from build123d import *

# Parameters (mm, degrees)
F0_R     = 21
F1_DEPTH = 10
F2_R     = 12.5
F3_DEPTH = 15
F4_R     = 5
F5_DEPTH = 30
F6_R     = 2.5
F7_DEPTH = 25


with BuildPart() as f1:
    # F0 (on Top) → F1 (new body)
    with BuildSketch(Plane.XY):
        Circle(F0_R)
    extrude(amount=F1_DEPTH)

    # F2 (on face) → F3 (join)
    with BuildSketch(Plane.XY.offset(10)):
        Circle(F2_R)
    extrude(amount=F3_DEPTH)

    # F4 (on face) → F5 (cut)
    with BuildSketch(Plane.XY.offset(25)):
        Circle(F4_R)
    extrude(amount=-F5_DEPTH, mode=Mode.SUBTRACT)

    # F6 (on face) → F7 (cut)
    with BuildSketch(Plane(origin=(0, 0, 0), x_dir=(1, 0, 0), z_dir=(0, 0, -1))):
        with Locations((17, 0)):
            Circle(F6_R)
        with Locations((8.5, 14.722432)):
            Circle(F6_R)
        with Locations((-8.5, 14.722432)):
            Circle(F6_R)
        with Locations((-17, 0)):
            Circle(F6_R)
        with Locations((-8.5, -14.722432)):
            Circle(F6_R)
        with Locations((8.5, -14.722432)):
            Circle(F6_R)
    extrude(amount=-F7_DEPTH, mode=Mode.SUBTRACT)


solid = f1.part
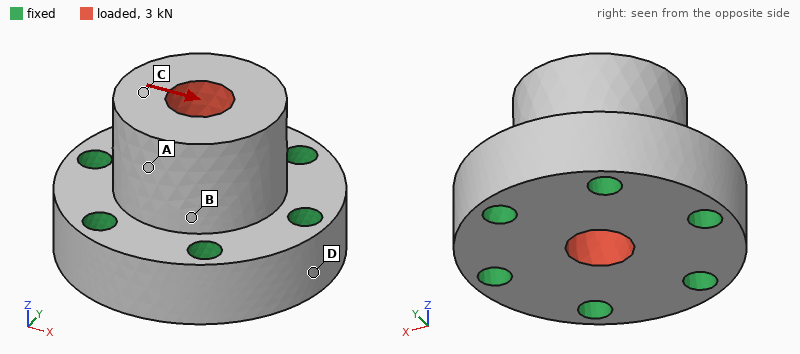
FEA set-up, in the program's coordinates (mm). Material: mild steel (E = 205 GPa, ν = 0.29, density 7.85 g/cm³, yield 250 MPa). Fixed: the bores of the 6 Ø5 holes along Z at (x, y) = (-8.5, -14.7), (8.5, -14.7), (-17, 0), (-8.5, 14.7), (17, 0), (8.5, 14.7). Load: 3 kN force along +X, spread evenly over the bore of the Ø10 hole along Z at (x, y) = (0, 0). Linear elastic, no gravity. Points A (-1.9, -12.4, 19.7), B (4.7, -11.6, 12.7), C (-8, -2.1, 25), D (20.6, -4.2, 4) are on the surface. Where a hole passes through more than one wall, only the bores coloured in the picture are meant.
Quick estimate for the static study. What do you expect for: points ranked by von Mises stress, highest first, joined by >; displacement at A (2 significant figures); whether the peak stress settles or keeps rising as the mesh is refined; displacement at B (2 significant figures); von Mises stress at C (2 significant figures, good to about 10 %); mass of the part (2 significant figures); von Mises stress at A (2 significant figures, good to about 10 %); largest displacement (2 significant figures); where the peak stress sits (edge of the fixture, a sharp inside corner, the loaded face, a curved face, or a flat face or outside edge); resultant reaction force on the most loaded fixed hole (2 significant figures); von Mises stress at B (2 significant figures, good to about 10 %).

B > C > A > D
0.98 µm
keeps rising
0.51 µm
5.3 MPa
140 g
2.9 MPa
1.6 µm
a sharp inside corner
880 N
7.3 MPa
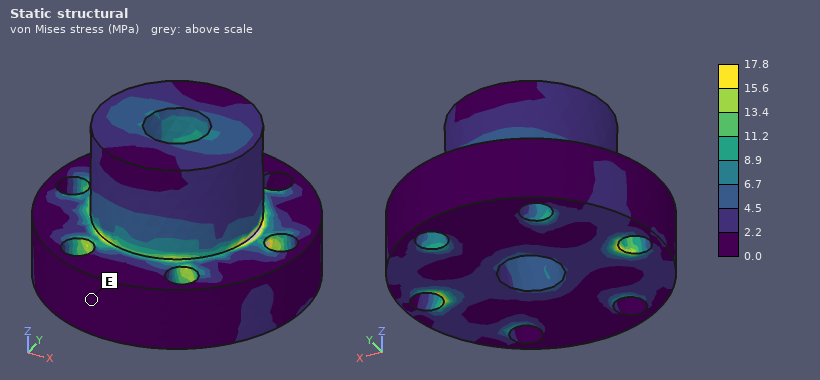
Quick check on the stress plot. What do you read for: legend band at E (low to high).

0.0 to 2.2 MPa
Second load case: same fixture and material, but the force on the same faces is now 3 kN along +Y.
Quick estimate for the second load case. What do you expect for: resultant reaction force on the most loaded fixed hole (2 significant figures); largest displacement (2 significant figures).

770 N
1.6 µm
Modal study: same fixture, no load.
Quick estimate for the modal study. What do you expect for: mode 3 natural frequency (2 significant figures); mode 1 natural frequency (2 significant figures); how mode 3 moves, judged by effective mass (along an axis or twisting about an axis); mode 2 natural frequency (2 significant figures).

43 kHz
29 kHz
along Z
29 kHz
